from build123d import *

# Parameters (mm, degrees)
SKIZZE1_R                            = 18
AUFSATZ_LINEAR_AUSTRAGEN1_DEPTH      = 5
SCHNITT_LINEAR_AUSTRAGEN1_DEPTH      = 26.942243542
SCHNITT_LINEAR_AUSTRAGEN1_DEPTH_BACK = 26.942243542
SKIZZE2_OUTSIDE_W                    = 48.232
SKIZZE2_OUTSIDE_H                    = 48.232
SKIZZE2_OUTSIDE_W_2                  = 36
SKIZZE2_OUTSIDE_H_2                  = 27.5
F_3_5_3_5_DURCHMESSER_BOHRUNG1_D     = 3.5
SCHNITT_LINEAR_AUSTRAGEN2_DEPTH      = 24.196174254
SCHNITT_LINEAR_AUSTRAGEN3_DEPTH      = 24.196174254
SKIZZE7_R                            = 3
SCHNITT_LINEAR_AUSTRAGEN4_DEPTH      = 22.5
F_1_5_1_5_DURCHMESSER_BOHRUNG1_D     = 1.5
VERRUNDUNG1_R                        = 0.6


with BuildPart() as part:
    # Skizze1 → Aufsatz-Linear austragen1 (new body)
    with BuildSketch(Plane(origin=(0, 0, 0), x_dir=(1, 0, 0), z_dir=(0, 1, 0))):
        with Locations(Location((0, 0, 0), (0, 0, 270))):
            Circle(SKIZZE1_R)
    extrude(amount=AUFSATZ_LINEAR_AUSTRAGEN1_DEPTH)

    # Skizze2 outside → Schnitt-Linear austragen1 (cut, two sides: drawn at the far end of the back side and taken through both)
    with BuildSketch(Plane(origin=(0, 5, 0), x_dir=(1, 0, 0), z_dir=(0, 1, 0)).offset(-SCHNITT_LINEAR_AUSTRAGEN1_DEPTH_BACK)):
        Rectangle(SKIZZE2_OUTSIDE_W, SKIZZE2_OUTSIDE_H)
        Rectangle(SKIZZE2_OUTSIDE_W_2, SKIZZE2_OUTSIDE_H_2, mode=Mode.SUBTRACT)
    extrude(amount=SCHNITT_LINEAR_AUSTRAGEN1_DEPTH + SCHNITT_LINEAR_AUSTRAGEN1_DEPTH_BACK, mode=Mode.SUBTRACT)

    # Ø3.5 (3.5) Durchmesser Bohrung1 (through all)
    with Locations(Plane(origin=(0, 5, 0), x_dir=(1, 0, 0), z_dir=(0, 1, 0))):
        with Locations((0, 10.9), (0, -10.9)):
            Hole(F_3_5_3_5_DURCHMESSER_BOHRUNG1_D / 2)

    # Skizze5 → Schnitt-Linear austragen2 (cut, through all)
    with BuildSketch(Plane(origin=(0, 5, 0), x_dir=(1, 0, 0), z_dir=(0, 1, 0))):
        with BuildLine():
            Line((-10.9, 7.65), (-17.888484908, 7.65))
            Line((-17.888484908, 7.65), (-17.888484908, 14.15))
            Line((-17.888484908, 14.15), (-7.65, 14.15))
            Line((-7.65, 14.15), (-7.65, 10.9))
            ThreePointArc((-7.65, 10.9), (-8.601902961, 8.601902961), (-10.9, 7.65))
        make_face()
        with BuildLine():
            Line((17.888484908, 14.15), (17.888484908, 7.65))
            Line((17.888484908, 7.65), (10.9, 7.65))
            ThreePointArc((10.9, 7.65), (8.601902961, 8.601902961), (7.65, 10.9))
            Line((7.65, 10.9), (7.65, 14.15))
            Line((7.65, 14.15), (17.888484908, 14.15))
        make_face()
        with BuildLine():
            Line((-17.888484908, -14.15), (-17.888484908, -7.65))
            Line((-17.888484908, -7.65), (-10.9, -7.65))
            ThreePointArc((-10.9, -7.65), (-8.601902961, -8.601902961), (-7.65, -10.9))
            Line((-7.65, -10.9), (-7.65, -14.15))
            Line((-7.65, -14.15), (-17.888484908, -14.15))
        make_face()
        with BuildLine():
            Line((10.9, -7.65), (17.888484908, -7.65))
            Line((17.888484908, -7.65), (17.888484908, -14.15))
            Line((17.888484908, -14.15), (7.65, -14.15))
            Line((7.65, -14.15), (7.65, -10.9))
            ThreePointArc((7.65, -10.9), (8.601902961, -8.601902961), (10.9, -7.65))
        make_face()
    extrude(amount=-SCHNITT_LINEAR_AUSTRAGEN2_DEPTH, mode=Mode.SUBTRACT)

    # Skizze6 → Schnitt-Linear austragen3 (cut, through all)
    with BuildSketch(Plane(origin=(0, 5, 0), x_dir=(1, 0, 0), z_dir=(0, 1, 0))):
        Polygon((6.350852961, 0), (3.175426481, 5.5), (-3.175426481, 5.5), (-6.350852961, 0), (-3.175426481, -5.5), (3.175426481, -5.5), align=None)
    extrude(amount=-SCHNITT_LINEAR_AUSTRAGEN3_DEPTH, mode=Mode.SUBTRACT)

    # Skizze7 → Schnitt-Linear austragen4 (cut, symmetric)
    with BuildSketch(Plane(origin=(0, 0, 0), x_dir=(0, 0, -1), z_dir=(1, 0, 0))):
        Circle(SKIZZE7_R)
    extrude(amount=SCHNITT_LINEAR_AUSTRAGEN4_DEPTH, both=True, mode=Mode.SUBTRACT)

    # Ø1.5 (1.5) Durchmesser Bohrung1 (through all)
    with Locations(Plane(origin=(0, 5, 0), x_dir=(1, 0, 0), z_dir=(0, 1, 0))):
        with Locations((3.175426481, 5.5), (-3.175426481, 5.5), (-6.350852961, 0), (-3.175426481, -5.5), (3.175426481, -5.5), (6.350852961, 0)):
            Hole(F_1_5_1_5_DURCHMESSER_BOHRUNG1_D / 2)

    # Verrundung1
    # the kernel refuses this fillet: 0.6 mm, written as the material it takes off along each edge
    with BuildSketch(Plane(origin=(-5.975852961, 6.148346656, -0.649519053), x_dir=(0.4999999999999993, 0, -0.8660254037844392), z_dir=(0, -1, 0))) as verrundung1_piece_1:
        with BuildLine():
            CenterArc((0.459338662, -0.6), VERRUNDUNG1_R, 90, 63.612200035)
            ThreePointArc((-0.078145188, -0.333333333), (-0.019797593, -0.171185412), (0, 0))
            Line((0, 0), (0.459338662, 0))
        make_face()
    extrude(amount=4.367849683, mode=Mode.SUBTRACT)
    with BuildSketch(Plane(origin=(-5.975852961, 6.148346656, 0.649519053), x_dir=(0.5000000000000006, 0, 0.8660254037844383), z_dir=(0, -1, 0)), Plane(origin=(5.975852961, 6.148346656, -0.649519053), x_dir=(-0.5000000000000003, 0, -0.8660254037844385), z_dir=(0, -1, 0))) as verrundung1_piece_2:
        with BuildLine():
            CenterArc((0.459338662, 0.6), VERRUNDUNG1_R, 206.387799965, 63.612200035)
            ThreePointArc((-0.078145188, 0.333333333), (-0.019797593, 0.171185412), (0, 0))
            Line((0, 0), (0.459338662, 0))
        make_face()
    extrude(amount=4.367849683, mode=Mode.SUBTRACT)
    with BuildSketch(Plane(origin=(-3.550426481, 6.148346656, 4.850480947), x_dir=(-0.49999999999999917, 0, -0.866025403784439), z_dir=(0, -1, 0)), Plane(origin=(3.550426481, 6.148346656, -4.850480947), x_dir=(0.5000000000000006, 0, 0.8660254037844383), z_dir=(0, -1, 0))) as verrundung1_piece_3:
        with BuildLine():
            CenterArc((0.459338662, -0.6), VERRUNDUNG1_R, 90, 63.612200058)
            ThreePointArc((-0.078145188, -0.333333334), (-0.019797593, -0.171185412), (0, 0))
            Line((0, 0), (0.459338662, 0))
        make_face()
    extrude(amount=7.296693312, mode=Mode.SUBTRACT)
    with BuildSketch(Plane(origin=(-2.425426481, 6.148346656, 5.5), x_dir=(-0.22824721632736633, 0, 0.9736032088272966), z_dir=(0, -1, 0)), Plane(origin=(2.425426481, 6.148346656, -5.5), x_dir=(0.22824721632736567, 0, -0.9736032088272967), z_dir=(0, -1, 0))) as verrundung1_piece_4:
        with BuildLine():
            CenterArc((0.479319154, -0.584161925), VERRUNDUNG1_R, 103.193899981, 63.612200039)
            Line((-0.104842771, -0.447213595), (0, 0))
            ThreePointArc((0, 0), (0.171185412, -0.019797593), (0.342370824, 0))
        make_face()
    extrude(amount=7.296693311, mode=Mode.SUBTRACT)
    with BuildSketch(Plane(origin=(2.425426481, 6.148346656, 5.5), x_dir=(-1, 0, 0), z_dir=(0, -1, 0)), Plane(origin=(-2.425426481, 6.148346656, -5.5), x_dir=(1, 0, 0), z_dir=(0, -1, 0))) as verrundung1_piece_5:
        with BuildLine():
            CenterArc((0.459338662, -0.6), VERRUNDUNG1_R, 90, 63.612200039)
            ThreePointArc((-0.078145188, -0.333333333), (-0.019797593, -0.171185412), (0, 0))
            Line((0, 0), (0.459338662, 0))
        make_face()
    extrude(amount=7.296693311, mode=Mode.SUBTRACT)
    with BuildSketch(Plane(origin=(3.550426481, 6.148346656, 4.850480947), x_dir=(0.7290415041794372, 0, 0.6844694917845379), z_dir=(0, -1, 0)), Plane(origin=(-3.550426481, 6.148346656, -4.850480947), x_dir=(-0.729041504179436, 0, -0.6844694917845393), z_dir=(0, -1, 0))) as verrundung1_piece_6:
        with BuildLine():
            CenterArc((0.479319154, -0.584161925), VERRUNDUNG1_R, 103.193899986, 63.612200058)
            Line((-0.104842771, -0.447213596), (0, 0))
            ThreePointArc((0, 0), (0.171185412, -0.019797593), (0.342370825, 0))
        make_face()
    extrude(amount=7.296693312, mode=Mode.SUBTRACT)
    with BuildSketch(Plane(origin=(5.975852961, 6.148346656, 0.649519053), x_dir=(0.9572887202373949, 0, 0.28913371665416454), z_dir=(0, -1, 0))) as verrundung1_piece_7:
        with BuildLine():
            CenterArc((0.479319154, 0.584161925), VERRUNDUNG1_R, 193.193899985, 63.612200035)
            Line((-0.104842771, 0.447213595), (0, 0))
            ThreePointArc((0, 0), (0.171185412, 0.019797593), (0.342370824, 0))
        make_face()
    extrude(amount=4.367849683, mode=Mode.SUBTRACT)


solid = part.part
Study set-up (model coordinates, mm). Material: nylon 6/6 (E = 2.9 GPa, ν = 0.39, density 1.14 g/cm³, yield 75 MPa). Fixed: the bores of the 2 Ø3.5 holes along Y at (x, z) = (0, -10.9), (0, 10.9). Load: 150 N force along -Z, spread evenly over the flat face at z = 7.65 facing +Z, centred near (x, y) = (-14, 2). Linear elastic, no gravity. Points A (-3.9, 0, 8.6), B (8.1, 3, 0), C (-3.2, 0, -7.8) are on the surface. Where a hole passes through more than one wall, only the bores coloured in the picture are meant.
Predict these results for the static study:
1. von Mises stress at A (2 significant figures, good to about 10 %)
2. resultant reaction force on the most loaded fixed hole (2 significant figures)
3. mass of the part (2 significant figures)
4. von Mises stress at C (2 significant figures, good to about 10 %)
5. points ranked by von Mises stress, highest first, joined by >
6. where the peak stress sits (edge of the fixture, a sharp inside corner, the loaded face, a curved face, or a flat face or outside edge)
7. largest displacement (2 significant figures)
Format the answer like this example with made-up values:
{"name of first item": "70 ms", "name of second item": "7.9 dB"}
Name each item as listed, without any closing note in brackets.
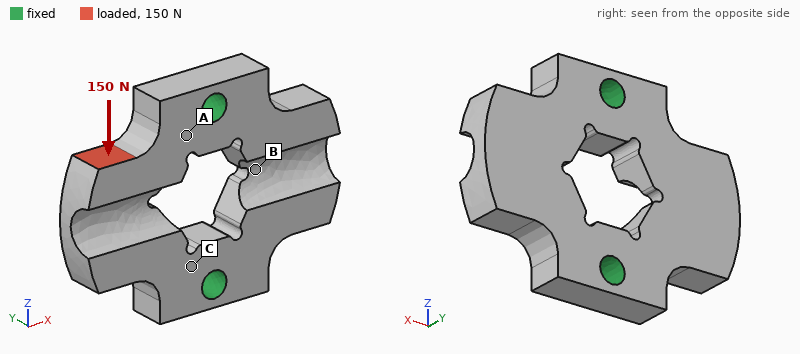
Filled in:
{"von Mises stress at A": "6.6 MPa", "resultant reaction force on the most loaded fixed hole": "110 N", "mass of the part": "3.0 g", "von Mises stress at C": "2.7 MPa", "points ranked by von Mises stress, highest first, joined by >": "A > C > B", "where the peak stress sits": "a curved face", "largest displacement": "93 µm"}
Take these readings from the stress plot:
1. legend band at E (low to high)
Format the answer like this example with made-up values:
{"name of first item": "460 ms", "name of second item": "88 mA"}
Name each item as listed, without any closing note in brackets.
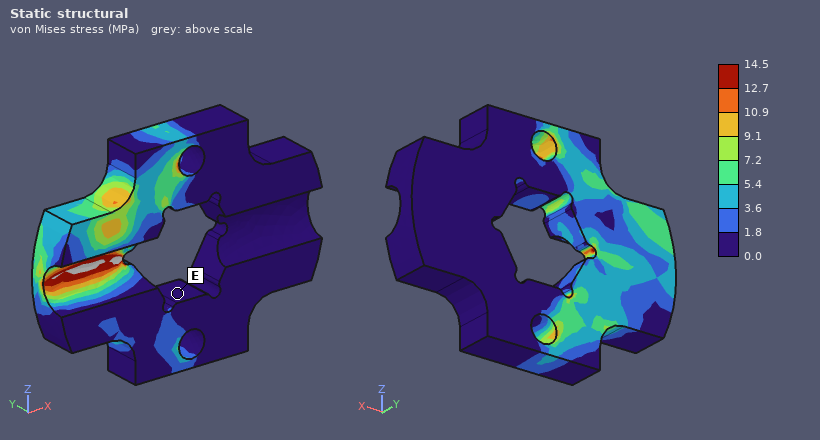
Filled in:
{"legend band at E": "0.0 to 1.8 MPa"}
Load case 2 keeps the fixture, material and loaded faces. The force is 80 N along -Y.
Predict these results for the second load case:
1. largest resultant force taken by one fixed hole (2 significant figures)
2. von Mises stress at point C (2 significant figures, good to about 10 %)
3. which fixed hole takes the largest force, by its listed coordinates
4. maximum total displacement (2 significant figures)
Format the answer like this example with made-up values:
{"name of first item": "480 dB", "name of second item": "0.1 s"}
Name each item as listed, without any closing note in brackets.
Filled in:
{"largest resultant force taken by one fixed hole": "68 N", "von Mises stress at point C": "10 MPa", "which fixed hole takes the largest force, by its listed coordinates": "(0, 10.9)", "maximum total displacement": "0.39 mm"}
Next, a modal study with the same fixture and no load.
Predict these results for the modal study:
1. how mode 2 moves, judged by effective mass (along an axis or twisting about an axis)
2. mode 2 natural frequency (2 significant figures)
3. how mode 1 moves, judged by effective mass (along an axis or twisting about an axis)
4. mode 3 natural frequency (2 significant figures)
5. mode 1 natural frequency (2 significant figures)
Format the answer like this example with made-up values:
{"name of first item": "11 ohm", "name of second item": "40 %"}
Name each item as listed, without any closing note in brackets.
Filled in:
{"how mode 2 moves, judged by effective mass": "along Y", "mode 2 natural frequency": "4000 Hz", "how mode 1 moves, judged by effective mass": "twisting about Z", "mode 3 natural frequency": "8500 Hz", "mode 1 natural frequency": "3800 Hz"}
